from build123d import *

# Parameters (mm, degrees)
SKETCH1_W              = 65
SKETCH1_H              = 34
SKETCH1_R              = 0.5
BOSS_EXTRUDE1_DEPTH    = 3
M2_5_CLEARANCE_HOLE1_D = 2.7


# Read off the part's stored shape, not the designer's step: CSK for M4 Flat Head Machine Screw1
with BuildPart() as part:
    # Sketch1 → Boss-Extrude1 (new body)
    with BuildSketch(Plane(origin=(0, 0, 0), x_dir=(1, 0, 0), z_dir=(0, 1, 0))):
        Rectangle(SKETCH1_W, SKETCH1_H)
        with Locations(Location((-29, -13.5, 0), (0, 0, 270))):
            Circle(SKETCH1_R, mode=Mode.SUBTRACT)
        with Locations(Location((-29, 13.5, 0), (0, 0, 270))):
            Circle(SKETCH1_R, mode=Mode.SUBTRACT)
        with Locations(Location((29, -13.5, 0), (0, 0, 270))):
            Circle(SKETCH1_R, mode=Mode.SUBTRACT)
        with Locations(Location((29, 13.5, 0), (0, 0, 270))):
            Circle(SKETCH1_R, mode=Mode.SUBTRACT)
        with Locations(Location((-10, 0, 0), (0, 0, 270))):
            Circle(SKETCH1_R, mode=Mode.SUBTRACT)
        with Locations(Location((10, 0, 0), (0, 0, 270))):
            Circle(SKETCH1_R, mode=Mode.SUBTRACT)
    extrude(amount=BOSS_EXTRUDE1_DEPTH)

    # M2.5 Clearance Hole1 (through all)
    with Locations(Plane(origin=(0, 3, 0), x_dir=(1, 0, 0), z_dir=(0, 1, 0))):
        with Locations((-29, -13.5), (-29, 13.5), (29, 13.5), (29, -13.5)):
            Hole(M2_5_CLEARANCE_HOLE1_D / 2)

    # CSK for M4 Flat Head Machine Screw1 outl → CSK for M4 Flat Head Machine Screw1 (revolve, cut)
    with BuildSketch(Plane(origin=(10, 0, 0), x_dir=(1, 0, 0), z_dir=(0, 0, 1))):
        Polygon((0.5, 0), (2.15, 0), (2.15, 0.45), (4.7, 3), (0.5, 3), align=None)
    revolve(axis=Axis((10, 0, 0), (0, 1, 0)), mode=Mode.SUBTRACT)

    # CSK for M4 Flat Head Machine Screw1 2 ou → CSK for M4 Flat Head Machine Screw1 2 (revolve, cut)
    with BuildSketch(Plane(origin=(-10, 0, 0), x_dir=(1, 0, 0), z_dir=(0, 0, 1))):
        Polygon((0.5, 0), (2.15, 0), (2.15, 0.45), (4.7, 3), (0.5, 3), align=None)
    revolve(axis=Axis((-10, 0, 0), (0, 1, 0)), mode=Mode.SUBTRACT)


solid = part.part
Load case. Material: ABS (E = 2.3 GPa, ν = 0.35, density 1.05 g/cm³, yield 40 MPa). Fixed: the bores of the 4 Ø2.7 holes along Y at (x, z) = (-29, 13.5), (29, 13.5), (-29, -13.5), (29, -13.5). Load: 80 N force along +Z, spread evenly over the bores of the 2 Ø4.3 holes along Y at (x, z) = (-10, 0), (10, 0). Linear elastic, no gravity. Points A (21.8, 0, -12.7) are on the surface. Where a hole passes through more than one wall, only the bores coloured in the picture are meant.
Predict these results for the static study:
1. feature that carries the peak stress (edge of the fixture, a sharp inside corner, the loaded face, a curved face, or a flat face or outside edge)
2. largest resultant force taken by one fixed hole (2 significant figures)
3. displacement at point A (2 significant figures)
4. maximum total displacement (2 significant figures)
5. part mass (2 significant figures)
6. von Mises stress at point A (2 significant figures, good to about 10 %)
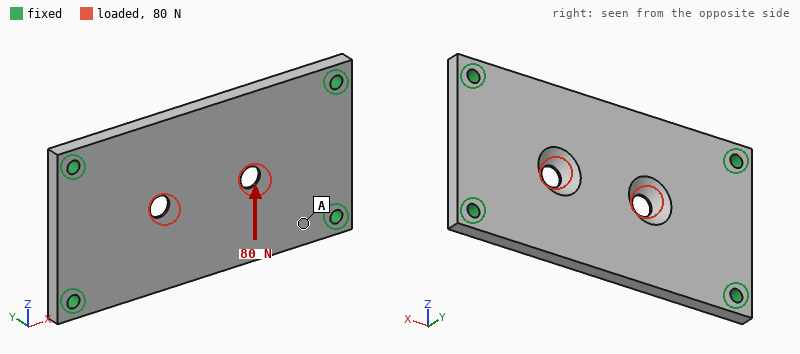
the loaded face
27 N
7.5 µm
36 µm
6.7 g
0.90 MPa
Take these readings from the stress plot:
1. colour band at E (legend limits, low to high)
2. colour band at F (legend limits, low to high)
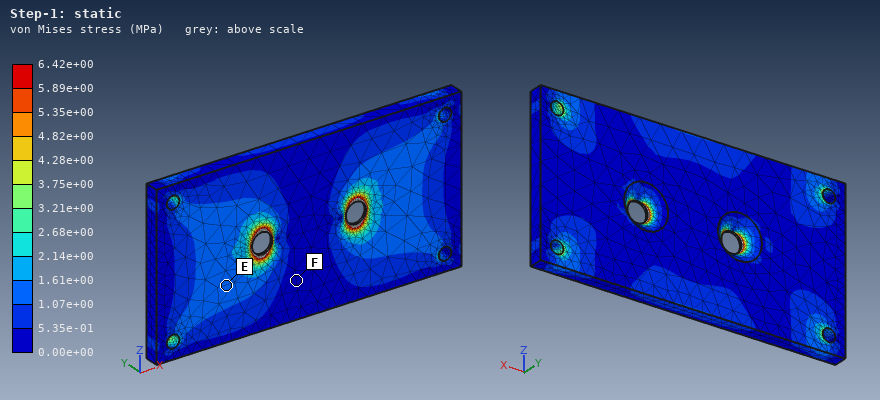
1.07e+00 to 1.61e+00 MPa
0.00e+00 to 5.35e-01 MPa
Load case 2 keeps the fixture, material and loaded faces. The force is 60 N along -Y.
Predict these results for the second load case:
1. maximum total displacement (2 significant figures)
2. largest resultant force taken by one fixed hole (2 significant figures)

0.36 mm
16 N
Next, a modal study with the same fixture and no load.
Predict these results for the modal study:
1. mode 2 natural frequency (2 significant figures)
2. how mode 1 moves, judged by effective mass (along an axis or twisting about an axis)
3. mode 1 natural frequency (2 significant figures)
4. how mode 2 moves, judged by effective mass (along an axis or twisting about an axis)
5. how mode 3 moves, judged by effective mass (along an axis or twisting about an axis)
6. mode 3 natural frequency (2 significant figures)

2000 Hz
along Y
1200 Hz
twisting about X
twisting about Z
3200 Hz
